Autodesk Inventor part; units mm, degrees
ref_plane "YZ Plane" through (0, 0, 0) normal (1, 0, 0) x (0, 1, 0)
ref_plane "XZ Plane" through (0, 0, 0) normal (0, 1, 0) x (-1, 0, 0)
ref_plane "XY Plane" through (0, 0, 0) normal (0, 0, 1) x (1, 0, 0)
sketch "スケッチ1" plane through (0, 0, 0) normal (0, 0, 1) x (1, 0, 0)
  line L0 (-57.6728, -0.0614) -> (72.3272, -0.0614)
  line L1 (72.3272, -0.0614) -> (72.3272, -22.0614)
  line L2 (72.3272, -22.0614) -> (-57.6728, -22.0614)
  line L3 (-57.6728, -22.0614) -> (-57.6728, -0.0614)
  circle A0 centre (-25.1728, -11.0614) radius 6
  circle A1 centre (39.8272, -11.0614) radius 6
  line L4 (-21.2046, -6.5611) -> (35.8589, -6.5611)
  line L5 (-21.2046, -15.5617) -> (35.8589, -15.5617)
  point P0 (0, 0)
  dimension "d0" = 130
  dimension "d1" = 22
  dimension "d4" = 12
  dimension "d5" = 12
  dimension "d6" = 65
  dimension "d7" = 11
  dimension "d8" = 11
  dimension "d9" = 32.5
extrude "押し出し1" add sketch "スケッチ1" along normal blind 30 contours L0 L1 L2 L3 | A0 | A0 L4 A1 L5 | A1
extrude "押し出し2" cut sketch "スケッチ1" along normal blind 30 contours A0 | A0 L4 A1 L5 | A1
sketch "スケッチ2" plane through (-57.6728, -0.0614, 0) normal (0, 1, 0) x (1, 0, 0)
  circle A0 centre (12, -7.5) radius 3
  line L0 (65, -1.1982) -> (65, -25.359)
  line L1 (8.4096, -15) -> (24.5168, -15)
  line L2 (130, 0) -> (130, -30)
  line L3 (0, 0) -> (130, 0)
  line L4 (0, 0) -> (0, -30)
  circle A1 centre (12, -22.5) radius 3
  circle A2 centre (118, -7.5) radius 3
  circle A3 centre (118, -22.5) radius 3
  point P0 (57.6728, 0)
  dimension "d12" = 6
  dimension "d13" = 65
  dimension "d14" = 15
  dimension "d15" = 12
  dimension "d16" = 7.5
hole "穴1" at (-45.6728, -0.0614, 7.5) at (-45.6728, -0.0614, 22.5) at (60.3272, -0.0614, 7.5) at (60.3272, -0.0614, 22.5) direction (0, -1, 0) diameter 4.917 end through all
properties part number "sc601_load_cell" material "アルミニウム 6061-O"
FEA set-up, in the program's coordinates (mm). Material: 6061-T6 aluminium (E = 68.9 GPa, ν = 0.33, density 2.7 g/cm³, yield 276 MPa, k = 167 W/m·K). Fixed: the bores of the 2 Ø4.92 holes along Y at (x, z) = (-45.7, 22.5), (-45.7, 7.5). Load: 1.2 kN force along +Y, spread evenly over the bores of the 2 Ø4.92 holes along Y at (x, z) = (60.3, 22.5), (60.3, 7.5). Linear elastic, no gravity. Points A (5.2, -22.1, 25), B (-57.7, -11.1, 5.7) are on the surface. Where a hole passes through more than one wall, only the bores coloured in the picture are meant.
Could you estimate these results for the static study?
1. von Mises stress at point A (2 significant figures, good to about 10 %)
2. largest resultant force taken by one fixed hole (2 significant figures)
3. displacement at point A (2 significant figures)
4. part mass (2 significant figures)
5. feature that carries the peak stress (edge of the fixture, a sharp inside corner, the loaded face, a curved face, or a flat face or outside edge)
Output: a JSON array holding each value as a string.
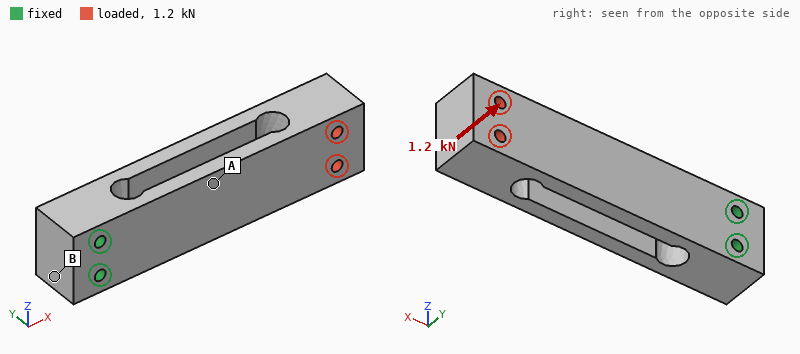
["38 MPa", "600 N", "0.40 mm", "170 g", "a curved face"]
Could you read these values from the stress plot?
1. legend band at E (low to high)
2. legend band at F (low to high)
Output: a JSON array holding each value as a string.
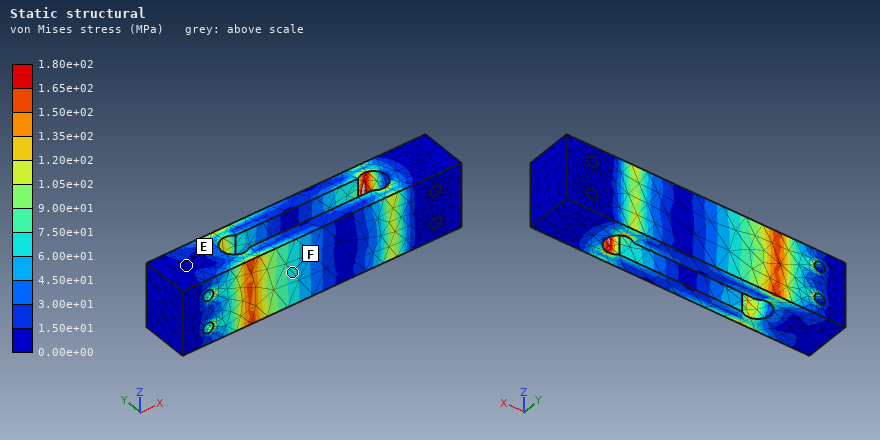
["0.00e+00 to 1.50e+01 MPa", "6.00e+01 to 7.50e+01 MPa"]
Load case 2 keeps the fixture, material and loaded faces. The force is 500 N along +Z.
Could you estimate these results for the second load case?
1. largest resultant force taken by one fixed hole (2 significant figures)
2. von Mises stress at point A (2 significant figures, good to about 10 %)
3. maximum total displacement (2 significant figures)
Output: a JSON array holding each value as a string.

["3.0 kN", "9.8 MPa", "0.12 mm"]
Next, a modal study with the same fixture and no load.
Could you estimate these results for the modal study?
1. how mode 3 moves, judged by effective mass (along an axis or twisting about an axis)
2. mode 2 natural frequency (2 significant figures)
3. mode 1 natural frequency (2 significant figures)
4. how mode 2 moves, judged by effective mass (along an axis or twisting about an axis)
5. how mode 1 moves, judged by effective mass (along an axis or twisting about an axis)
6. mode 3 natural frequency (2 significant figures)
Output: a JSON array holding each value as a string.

["twisting about X", "1400 Hz", "680 Hz", "along Z", "along Y", "2900 Hz"]
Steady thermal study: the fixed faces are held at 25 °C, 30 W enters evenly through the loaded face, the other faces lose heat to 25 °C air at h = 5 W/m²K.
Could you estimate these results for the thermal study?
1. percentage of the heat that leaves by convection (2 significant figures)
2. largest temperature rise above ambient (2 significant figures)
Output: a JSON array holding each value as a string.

["6.6 %", "44 K"]
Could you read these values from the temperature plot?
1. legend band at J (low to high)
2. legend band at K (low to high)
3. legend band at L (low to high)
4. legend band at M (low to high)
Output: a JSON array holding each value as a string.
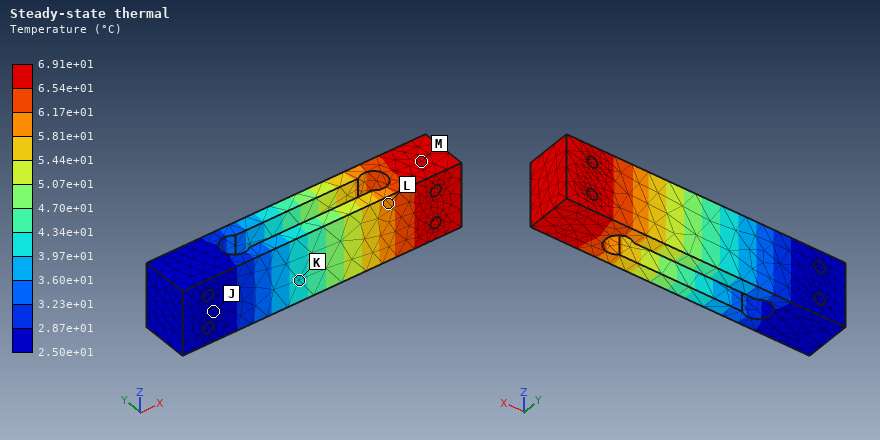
["2.50e+01 to 2.87e+01 °C", "3.97e+01 to 4.34e+01 °C", "5.81e+01 to 6.17e+01 °C", "6.54e+01 to 6.91e+01 °C"]
